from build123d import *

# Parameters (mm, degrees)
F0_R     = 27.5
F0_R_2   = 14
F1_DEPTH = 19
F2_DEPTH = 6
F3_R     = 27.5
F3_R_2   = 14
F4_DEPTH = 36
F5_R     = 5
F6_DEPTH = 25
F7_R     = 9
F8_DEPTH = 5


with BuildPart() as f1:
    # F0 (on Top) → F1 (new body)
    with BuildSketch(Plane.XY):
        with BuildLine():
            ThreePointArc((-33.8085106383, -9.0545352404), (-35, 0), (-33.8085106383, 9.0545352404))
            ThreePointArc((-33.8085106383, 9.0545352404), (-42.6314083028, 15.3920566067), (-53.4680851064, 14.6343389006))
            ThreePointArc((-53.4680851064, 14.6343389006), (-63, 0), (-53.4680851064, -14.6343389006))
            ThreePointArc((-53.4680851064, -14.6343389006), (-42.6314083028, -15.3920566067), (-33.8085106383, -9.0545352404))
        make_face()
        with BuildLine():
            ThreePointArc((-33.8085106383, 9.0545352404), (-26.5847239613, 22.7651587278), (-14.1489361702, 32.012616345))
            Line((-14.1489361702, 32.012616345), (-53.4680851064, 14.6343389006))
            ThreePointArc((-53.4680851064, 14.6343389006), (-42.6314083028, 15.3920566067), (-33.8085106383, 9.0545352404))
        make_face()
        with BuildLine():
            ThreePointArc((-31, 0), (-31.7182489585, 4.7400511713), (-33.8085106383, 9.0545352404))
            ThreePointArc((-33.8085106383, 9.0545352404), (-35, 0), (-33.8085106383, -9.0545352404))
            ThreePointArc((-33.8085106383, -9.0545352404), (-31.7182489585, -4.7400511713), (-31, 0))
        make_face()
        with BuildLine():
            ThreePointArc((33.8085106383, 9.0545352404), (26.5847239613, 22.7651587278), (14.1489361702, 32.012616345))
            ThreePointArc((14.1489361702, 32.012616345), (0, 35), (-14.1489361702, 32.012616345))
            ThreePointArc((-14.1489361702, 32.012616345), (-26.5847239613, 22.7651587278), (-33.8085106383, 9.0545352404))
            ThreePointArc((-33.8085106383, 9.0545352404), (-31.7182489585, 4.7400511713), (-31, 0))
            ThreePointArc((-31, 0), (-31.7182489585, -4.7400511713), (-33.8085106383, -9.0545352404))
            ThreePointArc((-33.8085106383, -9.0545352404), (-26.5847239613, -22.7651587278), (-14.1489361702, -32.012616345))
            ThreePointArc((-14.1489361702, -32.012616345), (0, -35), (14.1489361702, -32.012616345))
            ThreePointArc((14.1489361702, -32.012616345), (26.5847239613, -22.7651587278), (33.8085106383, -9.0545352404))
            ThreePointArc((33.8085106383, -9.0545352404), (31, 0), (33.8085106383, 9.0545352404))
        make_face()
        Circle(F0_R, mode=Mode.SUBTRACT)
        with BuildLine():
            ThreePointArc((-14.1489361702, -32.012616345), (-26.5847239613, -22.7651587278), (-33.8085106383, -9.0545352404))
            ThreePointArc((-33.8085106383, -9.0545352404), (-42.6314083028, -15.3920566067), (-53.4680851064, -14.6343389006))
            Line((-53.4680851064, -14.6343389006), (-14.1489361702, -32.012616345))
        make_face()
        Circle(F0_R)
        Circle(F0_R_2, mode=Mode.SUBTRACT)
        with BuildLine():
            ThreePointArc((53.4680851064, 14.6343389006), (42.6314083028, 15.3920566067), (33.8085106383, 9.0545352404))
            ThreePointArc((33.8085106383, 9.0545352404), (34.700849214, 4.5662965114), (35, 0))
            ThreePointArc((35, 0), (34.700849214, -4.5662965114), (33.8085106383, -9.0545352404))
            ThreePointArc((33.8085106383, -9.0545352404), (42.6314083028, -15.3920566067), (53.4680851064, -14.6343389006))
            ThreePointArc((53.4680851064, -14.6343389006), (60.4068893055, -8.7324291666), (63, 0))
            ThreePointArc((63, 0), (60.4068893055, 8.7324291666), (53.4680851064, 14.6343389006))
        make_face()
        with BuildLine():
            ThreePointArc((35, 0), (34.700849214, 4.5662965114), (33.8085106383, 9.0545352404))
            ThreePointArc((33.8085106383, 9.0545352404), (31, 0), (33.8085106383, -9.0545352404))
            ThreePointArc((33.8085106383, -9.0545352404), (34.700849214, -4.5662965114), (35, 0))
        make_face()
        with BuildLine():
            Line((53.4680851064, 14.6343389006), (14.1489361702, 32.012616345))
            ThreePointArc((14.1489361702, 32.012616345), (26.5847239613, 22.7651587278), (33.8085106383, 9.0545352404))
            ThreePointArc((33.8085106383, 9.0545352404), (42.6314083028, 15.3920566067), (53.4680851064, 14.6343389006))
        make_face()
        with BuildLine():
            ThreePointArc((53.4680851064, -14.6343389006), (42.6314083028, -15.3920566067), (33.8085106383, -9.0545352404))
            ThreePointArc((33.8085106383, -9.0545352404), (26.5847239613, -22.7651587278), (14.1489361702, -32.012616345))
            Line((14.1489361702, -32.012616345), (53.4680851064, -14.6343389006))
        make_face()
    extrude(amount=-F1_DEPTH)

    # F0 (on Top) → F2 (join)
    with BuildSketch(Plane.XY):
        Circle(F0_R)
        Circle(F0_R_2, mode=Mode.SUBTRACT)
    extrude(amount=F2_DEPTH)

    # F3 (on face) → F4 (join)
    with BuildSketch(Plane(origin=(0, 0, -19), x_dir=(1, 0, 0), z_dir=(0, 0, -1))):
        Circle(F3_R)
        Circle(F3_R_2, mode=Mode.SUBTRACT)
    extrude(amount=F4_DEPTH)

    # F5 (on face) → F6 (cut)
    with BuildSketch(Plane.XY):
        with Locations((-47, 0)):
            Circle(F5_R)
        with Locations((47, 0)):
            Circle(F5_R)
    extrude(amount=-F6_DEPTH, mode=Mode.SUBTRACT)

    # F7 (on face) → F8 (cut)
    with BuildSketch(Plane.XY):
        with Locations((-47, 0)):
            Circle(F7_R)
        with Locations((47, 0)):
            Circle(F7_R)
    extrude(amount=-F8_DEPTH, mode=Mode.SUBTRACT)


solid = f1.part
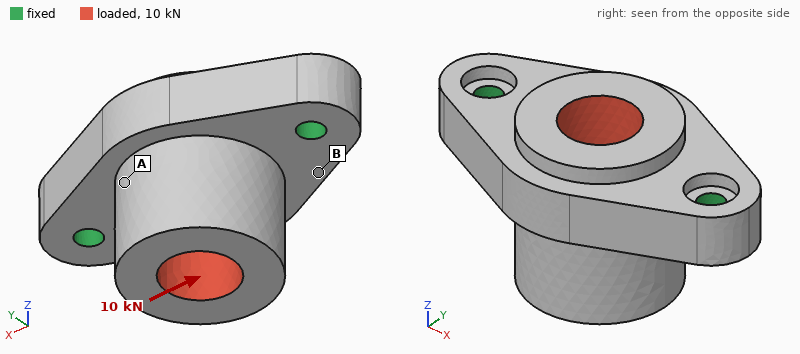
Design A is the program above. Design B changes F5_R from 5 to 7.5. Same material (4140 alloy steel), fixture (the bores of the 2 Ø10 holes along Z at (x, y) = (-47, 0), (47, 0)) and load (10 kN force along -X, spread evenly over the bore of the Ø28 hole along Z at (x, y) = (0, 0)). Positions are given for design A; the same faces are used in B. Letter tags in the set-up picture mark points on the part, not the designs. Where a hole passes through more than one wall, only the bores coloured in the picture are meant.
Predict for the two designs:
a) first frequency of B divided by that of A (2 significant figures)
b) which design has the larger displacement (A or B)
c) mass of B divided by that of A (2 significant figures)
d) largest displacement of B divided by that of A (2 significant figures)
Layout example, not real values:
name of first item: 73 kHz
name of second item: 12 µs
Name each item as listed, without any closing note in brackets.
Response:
first frequency of B divided by that of A: 1.2
which design has the larger displacement: A
mass of B divided by that of A: 0.98
largest displacement of B divided by that of A: 0.86
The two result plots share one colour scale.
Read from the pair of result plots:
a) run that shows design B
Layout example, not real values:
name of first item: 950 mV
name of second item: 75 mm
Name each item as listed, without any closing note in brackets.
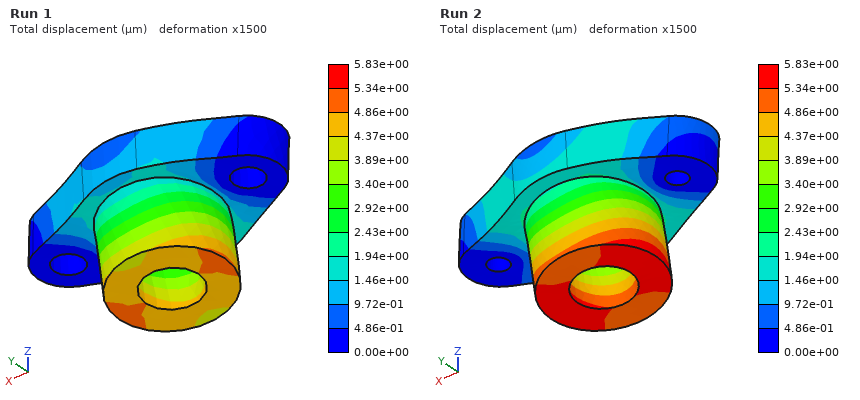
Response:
run that shows design B: Run 1
